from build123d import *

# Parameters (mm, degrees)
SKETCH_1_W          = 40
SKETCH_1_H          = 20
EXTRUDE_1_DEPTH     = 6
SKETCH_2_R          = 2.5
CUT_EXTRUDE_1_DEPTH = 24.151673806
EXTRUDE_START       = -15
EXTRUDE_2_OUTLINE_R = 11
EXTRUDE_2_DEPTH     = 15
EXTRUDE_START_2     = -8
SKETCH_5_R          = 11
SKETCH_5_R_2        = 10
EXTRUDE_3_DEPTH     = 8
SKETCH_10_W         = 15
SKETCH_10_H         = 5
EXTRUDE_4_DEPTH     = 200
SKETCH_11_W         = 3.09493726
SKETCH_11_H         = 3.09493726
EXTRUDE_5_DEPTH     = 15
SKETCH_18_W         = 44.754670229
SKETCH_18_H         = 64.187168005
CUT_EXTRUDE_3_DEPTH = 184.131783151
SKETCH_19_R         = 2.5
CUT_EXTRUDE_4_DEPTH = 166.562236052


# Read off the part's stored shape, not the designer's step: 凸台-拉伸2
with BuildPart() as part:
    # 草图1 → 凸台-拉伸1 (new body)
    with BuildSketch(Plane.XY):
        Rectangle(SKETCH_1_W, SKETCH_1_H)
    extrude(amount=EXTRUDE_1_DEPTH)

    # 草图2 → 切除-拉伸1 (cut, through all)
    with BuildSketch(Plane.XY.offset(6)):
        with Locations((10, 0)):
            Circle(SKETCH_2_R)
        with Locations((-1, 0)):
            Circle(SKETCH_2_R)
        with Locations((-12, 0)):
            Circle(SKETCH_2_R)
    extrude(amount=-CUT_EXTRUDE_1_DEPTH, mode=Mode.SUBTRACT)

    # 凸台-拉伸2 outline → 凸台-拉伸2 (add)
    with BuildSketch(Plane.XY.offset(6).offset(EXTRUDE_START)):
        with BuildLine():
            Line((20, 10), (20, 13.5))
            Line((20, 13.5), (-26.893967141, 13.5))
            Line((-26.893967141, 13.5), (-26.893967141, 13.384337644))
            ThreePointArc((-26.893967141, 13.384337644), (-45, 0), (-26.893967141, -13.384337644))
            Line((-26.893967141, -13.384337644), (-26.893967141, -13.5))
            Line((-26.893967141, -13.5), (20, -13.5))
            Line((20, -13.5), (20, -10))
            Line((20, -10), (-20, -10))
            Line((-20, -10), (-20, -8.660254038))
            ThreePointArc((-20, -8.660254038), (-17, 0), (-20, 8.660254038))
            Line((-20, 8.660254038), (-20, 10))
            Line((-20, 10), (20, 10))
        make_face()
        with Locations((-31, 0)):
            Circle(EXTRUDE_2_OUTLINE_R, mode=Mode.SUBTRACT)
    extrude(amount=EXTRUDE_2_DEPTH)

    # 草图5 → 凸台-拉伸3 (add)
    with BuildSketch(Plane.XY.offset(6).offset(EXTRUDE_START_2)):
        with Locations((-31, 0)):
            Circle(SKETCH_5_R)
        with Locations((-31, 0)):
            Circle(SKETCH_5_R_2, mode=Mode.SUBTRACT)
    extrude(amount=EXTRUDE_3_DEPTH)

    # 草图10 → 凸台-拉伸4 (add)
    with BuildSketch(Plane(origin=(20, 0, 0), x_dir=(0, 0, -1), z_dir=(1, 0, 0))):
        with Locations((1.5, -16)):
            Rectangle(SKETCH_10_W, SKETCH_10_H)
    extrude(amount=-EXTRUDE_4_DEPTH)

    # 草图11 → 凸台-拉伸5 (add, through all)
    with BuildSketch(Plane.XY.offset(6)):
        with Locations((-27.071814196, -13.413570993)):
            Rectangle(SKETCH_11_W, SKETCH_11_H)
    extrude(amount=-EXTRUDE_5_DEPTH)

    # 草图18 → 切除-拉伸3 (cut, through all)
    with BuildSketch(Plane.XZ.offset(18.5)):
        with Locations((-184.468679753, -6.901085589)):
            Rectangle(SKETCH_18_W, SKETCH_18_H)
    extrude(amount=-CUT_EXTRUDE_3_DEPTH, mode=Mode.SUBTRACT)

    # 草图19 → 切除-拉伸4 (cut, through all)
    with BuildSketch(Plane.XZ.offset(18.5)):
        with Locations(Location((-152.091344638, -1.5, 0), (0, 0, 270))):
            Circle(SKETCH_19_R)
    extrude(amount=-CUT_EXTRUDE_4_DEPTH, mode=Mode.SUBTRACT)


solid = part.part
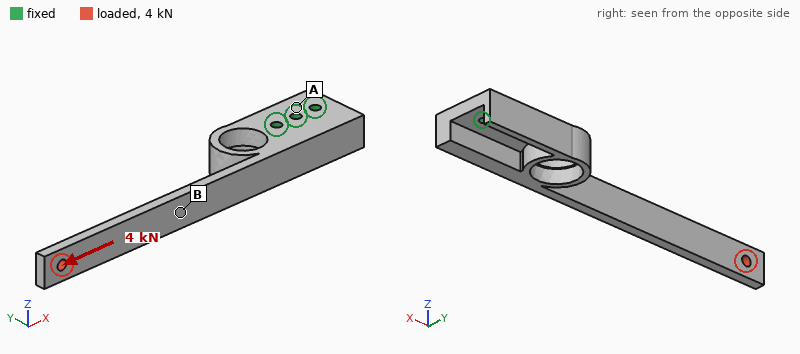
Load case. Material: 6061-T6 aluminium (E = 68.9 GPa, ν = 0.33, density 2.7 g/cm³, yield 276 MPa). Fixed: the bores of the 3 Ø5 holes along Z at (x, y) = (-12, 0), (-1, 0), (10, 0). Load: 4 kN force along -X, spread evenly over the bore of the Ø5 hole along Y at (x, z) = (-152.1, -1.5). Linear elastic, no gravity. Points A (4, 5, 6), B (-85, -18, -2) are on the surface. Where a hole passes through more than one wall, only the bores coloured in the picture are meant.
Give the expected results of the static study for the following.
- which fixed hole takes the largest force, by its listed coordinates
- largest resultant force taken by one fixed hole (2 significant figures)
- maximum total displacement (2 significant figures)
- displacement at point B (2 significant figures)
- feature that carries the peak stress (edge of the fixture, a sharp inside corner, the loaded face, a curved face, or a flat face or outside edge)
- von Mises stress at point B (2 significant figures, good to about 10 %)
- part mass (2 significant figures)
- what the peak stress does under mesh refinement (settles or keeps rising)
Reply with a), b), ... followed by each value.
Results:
a) (-12, 0)
b) 3.0 kN
c) 0.41 mm
d) 0.19 mm
e) edge of the fixture
f) 53 MPa
g) 71 g
h) keeps rising
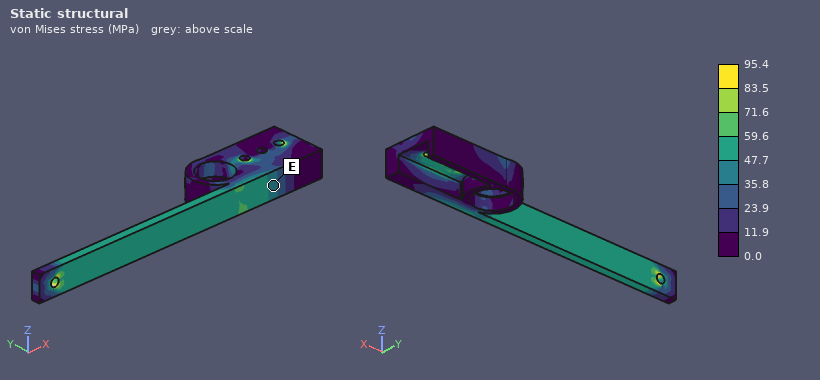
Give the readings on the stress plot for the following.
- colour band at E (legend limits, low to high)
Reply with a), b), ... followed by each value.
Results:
a) 35.8 to 47.7 MPa
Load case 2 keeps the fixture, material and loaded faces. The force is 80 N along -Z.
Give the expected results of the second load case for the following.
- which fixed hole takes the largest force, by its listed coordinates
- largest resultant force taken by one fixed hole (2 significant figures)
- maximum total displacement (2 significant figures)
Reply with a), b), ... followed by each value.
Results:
a) (-12, 0)
b) 490 N
c) 0.77 mm
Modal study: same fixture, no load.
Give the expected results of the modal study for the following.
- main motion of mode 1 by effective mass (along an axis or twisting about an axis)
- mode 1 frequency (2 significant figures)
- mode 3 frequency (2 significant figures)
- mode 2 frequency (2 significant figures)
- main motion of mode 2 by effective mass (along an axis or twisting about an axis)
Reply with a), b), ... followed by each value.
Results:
a) along Y
b) 240 Hz
c) 1500 Hz
d) 580 Hz
e) along Z
